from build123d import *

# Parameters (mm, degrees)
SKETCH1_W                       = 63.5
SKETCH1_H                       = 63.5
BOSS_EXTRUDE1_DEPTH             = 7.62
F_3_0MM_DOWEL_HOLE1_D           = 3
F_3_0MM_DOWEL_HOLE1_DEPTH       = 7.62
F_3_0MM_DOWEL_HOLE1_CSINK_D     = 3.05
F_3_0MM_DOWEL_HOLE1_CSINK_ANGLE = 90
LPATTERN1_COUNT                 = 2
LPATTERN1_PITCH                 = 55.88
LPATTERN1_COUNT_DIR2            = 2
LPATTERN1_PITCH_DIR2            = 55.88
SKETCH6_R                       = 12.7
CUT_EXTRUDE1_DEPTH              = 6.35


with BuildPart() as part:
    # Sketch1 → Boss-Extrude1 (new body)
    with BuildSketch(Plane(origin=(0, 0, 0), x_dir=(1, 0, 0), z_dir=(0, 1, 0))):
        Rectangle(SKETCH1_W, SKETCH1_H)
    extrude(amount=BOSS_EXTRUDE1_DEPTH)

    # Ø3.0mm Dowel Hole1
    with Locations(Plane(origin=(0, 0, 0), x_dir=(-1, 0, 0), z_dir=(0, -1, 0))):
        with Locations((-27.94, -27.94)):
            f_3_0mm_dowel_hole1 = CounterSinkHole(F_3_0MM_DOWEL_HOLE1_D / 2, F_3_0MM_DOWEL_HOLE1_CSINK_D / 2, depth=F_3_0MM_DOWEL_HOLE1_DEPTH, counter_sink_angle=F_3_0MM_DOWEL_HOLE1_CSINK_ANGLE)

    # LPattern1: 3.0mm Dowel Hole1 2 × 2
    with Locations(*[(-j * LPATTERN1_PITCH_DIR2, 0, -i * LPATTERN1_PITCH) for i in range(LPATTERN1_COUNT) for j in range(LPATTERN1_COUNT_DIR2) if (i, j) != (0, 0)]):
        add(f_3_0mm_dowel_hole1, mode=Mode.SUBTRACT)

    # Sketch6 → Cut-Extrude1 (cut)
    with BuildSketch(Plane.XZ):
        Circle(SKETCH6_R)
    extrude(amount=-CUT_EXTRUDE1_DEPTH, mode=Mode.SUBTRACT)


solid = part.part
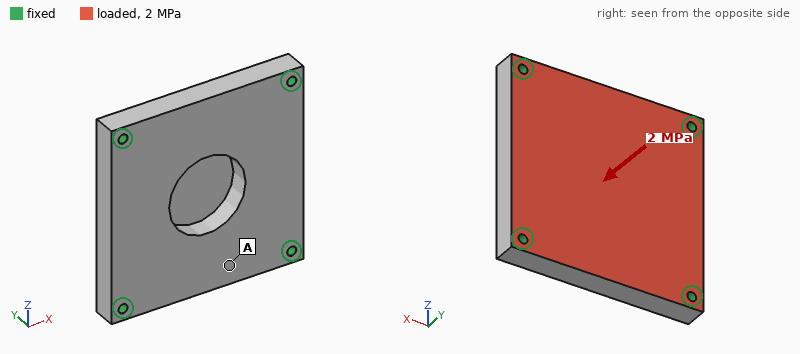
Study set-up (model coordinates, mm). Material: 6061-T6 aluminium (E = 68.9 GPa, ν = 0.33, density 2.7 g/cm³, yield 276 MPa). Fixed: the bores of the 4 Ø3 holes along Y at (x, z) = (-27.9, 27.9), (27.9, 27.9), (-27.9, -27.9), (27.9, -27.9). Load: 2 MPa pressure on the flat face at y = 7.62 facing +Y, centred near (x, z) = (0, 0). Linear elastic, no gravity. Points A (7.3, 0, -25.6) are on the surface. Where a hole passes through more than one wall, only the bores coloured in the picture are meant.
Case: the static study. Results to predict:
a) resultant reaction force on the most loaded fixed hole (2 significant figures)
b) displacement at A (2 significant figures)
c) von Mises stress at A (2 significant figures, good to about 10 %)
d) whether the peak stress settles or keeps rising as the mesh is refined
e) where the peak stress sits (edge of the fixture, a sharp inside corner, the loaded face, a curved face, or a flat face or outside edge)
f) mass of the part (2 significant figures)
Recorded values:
2.0 kN
0.047 mm
40 MPa
keeps rising
edge of the fixture
74 g
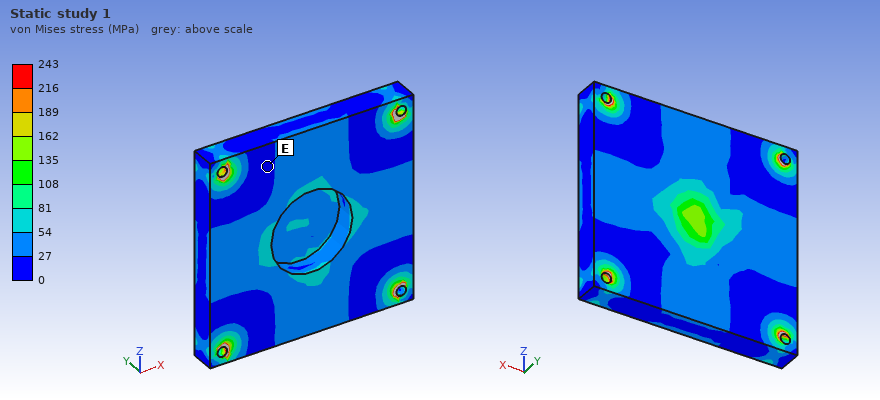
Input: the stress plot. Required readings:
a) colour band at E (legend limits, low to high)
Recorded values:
0 to 27 MPa
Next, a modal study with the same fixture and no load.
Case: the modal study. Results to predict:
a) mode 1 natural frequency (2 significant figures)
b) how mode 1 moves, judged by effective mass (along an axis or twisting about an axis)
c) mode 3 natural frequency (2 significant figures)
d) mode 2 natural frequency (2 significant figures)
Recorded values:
7300 Hz
along Y
11 kHz
11 kHz
